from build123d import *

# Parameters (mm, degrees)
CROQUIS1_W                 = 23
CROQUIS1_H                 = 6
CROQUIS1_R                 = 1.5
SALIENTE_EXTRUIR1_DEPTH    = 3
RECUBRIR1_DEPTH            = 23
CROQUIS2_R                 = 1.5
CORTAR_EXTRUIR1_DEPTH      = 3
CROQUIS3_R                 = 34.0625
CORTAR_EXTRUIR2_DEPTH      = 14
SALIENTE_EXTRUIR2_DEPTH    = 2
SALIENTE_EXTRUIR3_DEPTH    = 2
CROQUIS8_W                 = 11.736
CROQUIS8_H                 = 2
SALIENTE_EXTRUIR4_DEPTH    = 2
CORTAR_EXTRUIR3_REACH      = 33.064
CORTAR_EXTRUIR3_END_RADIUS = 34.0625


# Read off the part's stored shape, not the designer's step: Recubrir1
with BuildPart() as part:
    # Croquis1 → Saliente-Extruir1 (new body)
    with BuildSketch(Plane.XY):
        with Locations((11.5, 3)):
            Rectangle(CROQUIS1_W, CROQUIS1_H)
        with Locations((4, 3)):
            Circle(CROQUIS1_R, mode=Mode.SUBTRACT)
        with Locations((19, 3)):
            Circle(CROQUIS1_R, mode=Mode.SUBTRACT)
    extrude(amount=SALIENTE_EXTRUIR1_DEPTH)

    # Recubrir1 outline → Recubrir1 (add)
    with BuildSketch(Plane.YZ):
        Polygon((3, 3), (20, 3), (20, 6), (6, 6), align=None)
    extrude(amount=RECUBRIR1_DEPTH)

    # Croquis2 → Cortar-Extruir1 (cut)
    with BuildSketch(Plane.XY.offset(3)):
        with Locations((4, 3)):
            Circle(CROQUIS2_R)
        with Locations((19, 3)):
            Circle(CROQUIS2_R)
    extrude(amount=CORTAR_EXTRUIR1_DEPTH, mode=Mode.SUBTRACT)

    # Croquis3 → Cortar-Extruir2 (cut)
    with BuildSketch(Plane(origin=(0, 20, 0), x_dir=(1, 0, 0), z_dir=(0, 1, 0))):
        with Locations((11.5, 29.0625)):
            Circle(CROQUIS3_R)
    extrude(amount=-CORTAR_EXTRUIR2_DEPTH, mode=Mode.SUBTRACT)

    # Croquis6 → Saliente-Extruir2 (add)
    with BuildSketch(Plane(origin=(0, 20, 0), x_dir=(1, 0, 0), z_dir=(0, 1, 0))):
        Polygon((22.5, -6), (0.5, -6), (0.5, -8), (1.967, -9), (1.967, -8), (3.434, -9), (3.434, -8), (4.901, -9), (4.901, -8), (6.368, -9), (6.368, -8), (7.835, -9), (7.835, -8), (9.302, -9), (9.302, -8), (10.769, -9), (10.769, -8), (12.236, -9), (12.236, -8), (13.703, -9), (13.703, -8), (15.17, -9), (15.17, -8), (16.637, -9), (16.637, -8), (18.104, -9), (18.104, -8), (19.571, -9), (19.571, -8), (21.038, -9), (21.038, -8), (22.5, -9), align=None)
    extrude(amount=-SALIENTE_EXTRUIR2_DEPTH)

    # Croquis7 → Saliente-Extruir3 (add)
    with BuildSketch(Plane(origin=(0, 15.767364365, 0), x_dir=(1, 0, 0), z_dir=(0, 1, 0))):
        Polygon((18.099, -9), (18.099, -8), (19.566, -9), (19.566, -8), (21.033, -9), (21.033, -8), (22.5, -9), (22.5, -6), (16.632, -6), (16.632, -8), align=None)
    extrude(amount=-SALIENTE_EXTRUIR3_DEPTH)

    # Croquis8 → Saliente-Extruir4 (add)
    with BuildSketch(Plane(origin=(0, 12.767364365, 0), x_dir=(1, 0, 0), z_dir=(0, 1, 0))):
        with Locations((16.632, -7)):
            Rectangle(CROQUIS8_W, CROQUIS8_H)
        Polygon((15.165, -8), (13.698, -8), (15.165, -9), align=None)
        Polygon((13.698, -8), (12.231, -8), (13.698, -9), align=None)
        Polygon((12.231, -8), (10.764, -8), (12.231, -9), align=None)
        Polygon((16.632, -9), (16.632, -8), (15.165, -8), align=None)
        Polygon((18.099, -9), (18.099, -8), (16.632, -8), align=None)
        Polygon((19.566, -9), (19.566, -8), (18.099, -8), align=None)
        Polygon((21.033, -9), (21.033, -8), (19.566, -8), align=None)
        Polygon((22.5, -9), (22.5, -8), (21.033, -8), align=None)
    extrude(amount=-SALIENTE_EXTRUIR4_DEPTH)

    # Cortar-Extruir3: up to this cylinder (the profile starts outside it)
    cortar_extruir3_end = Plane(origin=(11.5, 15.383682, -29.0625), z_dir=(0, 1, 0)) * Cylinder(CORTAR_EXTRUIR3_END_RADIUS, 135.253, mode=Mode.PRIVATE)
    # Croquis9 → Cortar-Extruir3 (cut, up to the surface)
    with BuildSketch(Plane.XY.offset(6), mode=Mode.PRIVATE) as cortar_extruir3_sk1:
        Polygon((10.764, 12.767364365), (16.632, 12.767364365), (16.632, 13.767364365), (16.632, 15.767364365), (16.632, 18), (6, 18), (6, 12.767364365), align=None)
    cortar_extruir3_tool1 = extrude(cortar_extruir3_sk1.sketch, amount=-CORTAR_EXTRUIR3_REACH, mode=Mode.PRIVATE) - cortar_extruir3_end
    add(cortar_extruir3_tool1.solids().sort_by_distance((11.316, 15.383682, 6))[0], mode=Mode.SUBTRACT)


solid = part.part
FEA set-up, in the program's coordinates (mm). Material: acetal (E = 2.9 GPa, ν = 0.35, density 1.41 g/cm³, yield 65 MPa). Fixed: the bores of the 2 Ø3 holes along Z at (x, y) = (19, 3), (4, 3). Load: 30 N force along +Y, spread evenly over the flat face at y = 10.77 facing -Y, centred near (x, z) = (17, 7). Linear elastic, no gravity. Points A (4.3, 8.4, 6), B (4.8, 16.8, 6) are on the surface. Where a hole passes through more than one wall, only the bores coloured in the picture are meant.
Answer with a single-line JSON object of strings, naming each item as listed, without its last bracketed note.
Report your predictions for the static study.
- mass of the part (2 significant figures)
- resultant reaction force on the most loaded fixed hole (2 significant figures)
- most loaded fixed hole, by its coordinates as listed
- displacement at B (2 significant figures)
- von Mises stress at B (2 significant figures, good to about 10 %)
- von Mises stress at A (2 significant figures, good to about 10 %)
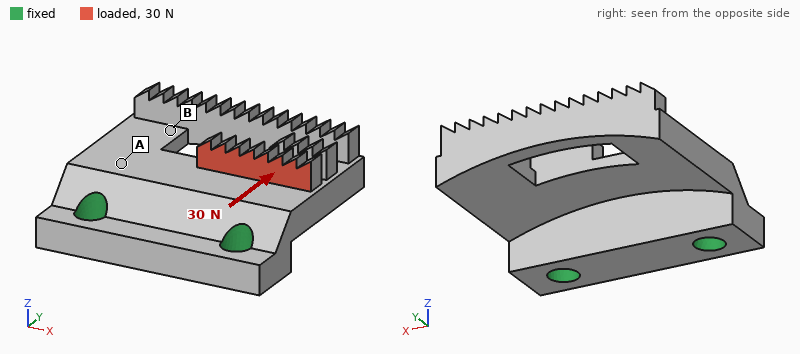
{"mass of the part": "1.6 g", "resultant reaction force on the most loaded fixed hole": "25 N", "most loaded fixed hole, by its coordinates as listed": "(19, 3)", "displacement at B": "0.12 mm", "von Mises stress at B": "1.3 MPa", "von Mises stress at A": "3.4 MPa"}
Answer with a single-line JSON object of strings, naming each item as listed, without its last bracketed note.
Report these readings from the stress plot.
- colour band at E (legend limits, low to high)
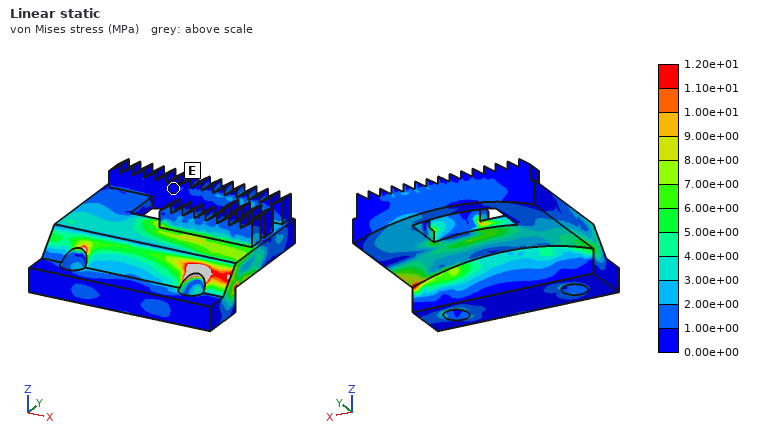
{"colour band at E": "0.00e+00 to 1.00e+00 MPa"}
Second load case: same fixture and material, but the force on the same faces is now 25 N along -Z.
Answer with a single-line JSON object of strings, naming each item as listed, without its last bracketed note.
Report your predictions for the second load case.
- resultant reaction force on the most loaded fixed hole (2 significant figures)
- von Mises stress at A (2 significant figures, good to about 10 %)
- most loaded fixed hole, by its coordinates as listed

{"resultant reaction force on the most loaded fixed hole": "20 N", "von Mises stress at A": "4.7 MPa", "most loaded fixed hole, by its coordinates as listed": "(19, 3)"}
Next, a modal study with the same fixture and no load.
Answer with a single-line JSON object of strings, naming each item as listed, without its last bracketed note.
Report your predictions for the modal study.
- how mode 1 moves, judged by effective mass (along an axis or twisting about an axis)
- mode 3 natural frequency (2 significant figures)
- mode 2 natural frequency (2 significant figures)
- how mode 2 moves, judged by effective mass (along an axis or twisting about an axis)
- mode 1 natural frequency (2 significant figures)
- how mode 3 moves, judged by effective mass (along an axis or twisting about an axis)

{"how mode 1 moves, judged by effective mass": "along Z", "mode 3 natural frequency": "5400 Hz", "mode 2 natural frequency": "2300 Hz", "how mode 2 moves, judged by effective mass": "twisting about Y", "mode 1 natural frequency": "1300 Hz", "how mode 3 moves, judged by effective mass": "along X"}
